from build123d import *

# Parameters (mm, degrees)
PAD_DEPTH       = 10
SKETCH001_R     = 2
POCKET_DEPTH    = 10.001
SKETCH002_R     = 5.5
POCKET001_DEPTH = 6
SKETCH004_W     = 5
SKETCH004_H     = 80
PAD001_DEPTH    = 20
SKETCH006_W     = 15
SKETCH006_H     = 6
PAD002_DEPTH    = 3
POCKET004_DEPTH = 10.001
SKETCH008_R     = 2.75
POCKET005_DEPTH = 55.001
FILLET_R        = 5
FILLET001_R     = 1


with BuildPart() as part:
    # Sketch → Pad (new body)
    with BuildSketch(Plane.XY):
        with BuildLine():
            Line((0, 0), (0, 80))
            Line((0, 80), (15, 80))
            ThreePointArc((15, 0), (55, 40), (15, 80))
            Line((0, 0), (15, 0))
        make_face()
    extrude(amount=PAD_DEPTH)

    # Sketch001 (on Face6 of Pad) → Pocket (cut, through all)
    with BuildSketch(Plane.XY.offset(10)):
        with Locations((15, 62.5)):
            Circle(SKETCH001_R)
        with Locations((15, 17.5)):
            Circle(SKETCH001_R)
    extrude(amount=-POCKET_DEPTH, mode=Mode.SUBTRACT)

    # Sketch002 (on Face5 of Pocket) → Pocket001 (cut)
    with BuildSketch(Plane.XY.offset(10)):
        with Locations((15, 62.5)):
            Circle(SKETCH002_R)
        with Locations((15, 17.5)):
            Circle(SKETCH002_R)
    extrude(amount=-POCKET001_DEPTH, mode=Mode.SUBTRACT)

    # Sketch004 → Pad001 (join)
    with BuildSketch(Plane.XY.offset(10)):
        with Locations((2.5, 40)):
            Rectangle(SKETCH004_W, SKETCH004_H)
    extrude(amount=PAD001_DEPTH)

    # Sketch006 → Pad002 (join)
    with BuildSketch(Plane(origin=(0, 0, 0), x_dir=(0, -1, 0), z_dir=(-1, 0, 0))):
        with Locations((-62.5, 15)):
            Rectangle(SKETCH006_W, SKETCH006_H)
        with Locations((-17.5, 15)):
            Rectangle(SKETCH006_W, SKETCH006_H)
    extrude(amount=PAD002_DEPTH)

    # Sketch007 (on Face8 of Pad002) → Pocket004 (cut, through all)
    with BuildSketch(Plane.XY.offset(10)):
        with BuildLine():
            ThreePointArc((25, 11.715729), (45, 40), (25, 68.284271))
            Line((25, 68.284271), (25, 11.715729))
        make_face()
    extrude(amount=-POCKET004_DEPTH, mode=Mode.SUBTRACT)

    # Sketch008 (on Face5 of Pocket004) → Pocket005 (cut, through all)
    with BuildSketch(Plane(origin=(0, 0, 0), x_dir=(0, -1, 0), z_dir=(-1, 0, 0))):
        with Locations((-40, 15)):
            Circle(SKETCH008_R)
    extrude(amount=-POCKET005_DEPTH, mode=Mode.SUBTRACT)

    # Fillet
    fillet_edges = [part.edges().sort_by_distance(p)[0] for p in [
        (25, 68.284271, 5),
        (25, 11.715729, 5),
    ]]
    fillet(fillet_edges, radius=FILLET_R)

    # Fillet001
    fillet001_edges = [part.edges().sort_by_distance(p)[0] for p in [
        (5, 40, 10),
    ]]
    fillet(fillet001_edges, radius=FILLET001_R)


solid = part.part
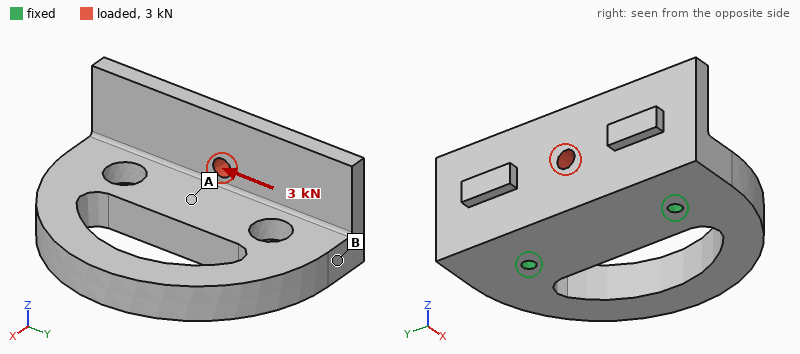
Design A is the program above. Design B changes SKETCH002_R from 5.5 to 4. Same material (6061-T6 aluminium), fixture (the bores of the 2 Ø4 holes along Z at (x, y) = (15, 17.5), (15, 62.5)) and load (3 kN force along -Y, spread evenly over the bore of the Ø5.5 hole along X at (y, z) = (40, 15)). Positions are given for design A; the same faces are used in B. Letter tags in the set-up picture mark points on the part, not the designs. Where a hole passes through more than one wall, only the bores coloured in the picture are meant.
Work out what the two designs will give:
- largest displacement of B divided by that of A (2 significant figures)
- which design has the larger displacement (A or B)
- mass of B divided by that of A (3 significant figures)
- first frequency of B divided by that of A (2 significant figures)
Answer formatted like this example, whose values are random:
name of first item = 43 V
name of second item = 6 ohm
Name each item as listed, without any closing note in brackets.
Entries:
largest displacement of B divided by that of A = 0.91
which design has the larger displacement = A
mass of B divided by that of A = 1.01
first frequency of B divided by that of A = 1.0
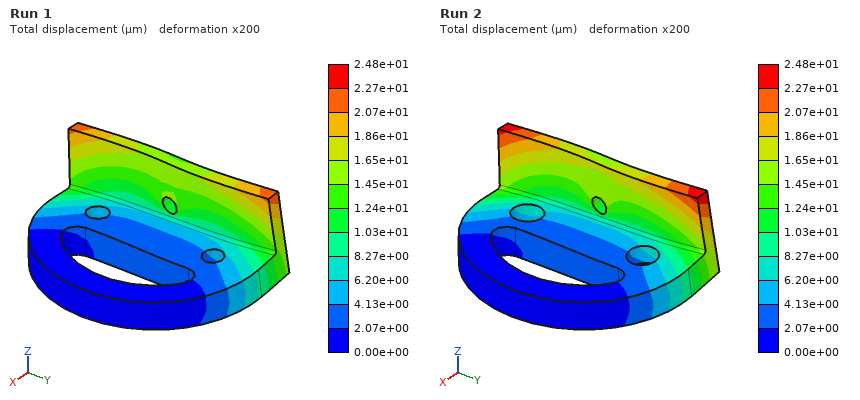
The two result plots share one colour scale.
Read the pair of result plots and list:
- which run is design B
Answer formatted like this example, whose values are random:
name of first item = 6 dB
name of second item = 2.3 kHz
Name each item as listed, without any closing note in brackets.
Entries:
which run is design B = Run 1
